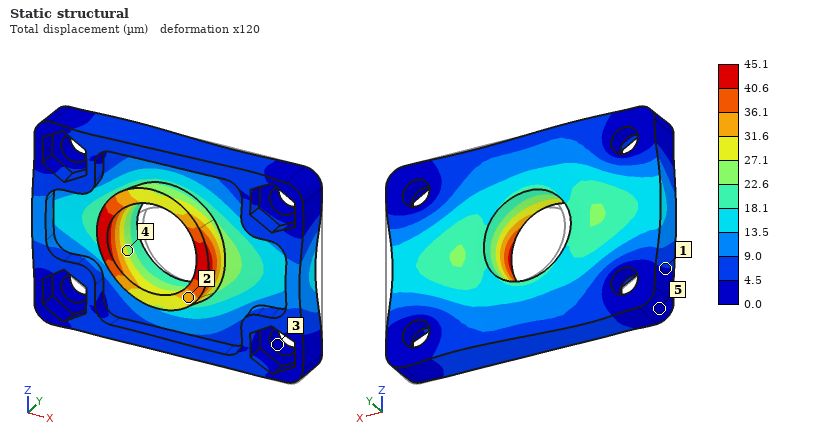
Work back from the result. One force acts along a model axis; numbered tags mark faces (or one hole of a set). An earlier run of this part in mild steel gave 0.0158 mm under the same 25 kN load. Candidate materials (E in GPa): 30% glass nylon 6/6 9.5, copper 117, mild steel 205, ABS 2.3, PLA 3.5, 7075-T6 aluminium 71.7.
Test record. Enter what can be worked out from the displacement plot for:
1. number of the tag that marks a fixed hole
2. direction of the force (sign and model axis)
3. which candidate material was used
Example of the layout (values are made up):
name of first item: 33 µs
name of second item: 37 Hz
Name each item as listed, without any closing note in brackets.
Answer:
number of the tag that marks a fixed hole: 3
direction of the force: -X
which candidate material was used: 7075-T6 aluminium
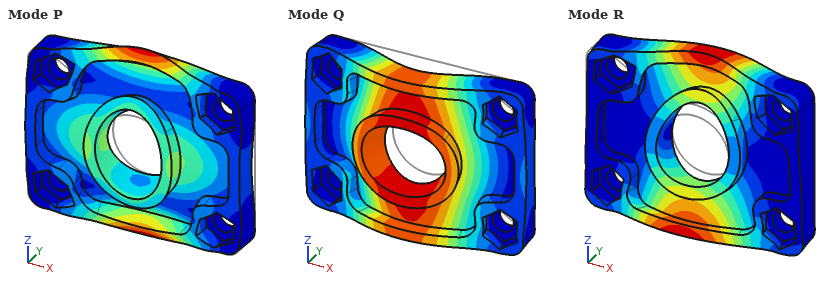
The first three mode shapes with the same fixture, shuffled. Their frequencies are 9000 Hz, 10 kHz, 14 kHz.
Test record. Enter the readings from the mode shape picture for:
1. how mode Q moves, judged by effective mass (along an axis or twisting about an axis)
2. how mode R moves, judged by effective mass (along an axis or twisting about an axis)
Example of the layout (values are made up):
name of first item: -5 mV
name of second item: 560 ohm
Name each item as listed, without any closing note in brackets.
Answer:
how mode Q moves, judged by effective mass: along Y
how mode R moves, judged by effective mass: twisting about X
